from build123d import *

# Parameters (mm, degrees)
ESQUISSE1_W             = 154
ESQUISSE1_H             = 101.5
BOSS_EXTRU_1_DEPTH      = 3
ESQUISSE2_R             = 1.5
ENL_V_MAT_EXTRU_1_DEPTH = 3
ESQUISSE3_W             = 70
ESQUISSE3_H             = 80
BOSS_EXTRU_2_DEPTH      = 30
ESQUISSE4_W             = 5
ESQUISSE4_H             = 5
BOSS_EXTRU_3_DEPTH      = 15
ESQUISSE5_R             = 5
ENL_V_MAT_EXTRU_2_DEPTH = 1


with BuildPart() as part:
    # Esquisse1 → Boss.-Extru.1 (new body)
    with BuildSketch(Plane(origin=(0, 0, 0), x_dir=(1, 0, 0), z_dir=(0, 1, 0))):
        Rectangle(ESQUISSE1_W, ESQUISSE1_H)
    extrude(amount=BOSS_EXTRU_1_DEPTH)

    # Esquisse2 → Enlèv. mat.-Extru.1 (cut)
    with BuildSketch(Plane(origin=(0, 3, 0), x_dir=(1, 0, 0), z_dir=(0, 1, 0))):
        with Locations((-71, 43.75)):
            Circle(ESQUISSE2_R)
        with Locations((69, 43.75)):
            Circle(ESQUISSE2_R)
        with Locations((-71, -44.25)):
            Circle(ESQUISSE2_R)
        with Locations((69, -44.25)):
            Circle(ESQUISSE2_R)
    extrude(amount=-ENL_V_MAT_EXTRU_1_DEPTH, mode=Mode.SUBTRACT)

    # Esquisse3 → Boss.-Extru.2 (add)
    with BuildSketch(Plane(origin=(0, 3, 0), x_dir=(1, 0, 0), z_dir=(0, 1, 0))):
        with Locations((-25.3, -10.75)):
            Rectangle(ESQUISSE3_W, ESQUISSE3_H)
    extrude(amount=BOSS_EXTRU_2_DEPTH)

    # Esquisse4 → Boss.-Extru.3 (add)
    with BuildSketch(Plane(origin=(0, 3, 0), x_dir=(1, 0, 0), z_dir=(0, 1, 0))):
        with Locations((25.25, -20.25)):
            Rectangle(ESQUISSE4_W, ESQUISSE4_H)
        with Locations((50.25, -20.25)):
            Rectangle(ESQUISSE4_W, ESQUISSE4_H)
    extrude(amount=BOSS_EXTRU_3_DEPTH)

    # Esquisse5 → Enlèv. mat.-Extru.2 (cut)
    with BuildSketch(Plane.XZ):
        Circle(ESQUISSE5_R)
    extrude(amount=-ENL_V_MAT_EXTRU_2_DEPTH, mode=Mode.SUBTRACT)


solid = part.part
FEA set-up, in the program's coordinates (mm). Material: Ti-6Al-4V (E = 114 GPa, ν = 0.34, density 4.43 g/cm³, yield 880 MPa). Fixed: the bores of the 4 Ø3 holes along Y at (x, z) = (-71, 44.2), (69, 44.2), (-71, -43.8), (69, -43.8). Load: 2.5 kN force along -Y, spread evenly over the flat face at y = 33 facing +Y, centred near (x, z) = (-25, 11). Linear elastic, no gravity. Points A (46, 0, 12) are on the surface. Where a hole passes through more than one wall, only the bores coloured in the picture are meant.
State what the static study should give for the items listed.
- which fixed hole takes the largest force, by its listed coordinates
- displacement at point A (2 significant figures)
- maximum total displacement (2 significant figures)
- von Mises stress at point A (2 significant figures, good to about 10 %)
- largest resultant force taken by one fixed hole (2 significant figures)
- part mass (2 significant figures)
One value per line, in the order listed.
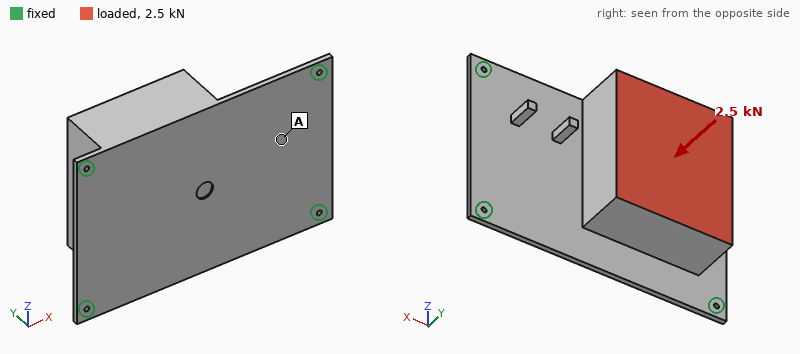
(-71, 44.2)
0.39 mm
0.69 mm
34 MPa
1.2 kN
950 g
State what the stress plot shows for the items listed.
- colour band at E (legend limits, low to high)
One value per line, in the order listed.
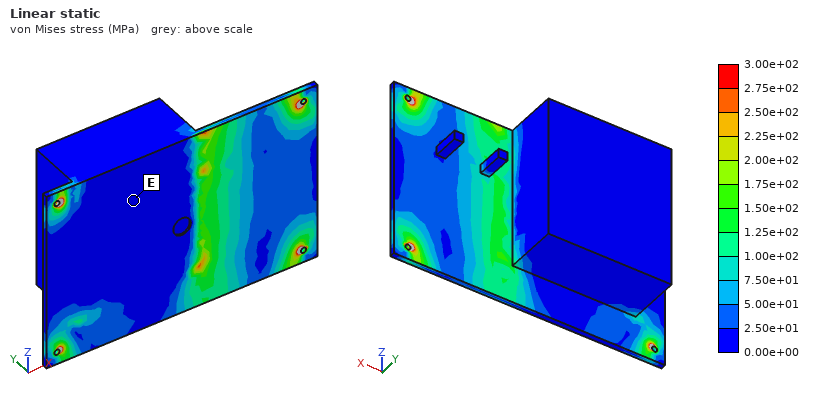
0.00e+00 to 2.50e+01 MPa
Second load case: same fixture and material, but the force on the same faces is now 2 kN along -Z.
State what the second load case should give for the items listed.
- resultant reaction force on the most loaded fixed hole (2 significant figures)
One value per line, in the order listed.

1.2 kN
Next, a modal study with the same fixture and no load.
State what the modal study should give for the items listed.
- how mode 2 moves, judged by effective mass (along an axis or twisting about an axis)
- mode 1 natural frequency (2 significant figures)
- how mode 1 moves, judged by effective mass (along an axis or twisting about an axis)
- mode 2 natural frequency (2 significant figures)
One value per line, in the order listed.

along Z
370 Hz
along Y
1000 Hz
